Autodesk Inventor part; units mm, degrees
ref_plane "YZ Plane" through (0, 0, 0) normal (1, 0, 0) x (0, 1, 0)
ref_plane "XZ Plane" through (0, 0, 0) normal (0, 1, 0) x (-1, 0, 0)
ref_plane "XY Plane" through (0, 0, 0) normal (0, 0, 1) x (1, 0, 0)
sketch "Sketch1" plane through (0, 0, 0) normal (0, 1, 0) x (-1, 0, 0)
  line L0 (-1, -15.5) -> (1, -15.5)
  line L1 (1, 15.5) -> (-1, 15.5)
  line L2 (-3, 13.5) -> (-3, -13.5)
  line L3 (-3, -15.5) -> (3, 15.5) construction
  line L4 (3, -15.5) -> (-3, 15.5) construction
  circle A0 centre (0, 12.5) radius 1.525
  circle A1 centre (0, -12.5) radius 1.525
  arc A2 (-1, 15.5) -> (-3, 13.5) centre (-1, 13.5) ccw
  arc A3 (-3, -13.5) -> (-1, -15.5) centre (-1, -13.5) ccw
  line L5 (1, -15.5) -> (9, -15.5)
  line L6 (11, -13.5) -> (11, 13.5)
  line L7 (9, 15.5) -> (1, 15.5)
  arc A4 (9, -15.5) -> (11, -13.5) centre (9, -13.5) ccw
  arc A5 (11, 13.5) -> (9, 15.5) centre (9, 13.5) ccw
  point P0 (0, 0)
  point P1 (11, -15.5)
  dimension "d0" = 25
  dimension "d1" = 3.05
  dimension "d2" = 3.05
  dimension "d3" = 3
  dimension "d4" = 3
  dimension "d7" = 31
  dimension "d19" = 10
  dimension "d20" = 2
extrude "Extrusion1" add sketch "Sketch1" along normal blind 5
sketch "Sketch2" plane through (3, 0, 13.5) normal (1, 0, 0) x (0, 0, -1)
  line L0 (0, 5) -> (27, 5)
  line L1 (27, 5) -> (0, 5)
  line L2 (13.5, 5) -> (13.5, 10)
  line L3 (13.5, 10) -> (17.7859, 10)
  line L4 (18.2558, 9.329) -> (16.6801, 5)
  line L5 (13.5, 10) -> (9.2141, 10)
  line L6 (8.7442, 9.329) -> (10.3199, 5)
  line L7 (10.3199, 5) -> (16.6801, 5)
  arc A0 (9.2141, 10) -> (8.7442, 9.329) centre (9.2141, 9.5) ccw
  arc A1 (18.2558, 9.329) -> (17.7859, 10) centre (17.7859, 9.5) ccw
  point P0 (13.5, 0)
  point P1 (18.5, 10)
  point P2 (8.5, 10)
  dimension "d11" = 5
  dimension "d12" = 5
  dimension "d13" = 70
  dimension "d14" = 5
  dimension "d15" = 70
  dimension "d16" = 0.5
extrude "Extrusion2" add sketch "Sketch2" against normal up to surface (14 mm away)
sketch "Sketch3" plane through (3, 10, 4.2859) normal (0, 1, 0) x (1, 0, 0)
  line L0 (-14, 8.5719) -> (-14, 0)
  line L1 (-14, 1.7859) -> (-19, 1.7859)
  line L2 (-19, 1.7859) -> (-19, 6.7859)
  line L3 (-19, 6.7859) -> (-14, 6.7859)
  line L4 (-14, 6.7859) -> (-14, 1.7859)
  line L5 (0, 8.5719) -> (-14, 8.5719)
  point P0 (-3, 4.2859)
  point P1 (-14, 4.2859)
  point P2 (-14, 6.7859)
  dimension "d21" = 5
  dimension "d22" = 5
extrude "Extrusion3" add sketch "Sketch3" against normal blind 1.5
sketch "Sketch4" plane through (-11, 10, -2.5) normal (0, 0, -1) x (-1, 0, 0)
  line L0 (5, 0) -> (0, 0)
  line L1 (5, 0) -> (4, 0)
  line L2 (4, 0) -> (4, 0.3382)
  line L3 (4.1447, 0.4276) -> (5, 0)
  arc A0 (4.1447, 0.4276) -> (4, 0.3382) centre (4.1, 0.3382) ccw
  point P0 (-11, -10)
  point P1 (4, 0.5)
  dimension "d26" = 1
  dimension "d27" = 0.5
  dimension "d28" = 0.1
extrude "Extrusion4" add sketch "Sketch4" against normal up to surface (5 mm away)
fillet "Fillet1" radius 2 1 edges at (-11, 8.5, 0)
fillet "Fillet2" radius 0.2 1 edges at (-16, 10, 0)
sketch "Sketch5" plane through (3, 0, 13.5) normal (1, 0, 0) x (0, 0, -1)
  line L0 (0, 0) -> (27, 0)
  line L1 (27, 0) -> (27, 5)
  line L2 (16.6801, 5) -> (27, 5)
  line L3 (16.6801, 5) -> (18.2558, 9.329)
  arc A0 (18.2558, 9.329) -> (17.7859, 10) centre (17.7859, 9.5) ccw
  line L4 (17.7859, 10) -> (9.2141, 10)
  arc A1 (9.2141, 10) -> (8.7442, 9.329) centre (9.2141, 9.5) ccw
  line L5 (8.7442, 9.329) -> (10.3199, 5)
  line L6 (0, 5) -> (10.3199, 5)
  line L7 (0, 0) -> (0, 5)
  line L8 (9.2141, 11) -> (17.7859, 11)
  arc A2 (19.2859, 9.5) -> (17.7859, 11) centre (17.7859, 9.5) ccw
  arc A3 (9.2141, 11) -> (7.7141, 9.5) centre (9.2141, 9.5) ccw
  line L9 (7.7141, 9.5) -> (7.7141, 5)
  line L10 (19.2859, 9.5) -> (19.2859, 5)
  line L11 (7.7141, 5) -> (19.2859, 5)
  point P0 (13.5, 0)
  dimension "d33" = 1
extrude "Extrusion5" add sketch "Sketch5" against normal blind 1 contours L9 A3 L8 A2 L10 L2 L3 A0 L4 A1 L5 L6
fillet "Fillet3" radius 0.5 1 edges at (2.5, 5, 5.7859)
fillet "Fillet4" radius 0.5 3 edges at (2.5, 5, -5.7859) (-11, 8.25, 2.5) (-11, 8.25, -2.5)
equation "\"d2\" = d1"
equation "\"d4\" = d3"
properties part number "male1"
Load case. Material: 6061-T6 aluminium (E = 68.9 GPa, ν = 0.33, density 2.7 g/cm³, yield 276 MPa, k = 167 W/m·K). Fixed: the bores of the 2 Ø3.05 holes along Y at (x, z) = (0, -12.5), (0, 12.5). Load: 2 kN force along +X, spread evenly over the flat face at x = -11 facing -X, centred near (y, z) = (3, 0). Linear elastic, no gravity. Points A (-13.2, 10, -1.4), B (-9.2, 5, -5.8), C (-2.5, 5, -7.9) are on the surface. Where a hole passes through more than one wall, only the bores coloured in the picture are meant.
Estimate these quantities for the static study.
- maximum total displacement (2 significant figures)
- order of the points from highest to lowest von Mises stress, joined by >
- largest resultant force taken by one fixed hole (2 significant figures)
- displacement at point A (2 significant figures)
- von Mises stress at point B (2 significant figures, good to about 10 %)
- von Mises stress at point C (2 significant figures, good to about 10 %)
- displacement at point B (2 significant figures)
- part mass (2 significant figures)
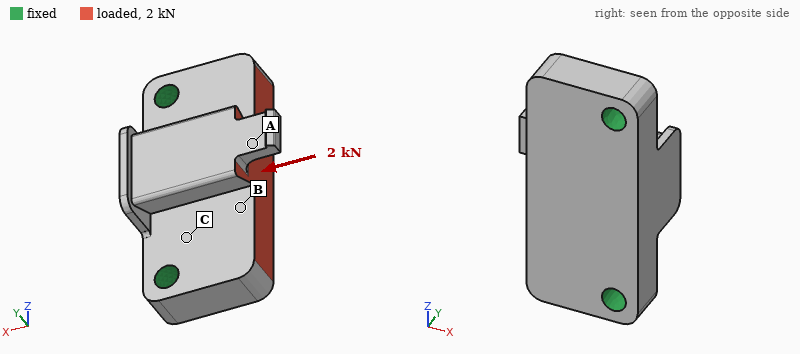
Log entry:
14 µm
C > B > A
1.1 kN
13 µm
19 MPa
36 MPa
7.8 µm
7.3 g
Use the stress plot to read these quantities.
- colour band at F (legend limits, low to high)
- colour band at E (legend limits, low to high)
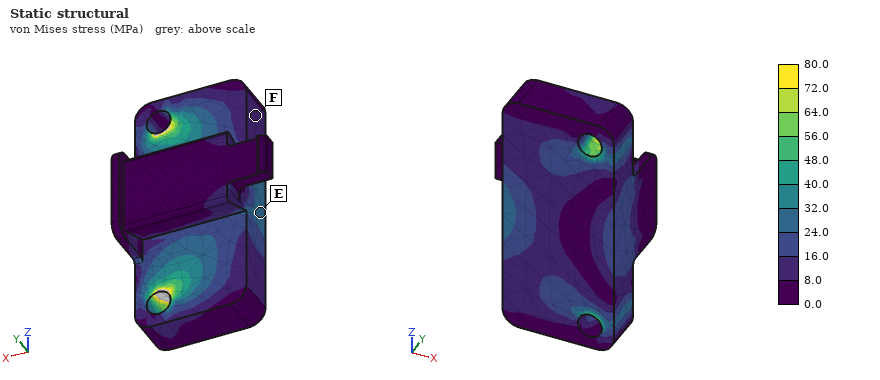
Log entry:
8.0 to 16.0 MPa
24.0 to 32.0 MPa
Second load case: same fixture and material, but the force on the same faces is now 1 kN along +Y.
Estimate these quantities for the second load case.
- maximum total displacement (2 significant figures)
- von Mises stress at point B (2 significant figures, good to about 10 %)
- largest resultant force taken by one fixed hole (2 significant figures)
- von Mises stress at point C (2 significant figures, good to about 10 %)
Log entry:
69 µm
34 MPa
500 N
60 MPa
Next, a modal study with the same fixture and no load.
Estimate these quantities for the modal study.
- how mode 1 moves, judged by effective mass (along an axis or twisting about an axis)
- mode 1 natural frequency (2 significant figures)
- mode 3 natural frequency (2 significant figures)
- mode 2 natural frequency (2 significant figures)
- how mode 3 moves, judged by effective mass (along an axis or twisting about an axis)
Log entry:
along Y
15 kHz
34 kHz
28 kHz
along Z
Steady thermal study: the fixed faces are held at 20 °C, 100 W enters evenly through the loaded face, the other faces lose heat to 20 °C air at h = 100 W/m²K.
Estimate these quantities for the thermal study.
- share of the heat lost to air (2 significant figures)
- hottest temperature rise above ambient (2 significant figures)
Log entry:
4.4 %
58 K
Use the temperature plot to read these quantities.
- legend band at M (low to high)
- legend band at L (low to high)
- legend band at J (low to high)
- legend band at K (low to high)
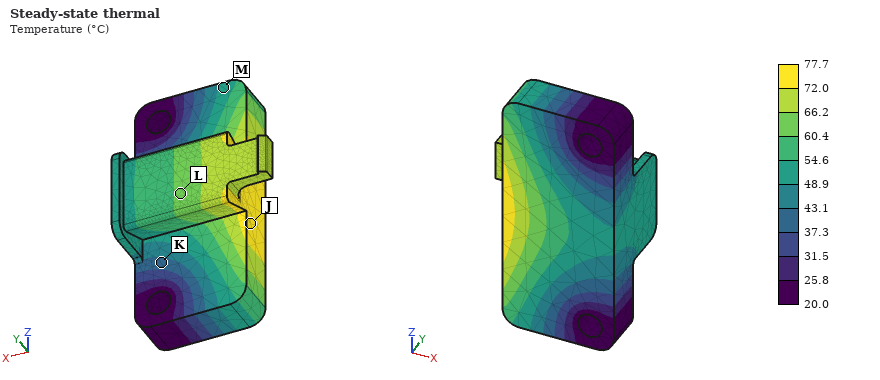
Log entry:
48.9 to 54.6 °C
60.4 to 66.2 °C
72.0 to 77.7 °C
37.3 to 43.1 °C
